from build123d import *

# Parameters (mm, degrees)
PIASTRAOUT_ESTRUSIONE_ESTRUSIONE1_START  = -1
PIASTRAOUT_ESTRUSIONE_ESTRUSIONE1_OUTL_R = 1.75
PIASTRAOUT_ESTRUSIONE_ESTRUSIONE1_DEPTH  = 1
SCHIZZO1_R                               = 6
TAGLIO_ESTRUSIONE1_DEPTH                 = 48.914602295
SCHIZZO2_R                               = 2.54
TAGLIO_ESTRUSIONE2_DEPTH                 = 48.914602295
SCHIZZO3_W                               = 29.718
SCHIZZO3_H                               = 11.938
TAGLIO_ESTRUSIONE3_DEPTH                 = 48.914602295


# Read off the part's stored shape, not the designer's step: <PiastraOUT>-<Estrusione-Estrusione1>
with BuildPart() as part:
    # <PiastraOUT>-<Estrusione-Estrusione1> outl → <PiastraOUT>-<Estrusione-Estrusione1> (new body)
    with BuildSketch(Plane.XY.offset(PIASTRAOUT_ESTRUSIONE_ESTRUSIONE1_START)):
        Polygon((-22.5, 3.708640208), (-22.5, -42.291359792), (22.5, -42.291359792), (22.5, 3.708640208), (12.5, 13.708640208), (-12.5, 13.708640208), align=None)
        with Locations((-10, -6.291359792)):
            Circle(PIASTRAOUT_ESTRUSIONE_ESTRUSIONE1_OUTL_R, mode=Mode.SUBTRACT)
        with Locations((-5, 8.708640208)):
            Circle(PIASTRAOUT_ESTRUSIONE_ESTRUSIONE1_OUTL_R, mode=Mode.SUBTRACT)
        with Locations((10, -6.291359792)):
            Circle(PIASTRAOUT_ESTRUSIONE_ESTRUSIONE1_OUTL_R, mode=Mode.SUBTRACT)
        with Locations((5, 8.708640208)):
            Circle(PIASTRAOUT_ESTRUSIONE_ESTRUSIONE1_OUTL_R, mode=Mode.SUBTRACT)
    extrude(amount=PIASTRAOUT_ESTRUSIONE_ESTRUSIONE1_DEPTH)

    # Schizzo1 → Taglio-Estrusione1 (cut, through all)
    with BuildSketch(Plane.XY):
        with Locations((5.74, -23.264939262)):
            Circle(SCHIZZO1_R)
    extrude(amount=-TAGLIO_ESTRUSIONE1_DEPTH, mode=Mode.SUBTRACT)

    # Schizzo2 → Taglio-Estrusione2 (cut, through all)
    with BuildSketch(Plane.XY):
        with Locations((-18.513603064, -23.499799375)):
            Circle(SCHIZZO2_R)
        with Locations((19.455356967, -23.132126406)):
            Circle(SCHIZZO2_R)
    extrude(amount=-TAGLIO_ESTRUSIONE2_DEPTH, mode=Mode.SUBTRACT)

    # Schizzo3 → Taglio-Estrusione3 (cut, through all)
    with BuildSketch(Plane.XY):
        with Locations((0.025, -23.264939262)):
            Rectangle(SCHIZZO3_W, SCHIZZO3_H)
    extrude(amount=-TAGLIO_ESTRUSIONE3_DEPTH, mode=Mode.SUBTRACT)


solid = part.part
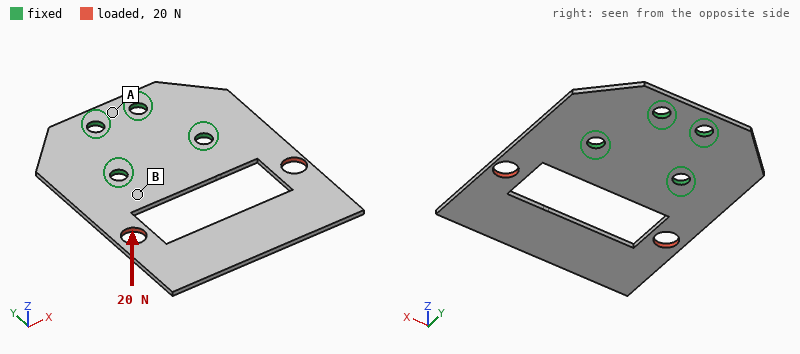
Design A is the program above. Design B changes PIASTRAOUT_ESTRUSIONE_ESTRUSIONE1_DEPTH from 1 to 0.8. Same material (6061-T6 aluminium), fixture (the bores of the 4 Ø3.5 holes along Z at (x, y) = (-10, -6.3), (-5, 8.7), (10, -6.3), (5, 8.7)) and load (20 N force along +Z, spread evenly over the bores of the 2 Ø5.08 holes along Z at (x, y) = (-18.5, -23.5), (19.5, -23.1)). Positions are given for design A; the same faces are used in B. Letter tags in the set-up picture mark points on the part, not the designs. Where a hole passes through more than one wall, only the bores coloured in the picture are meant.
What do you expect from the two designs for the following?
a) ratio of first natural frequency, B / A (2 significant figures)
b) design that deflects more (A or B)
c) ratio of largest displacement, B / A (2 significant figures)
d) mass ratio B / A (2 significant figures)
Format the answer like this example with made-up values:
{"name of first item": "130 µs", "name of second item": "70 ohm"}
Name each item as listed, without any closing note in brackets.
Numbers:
{"ratio of first natural frequency, B / A": "0.80", "design that deflects more": "B", "ratio of largest displacement, B / A": "1.9", "mass ratio B / A": "0.80"}
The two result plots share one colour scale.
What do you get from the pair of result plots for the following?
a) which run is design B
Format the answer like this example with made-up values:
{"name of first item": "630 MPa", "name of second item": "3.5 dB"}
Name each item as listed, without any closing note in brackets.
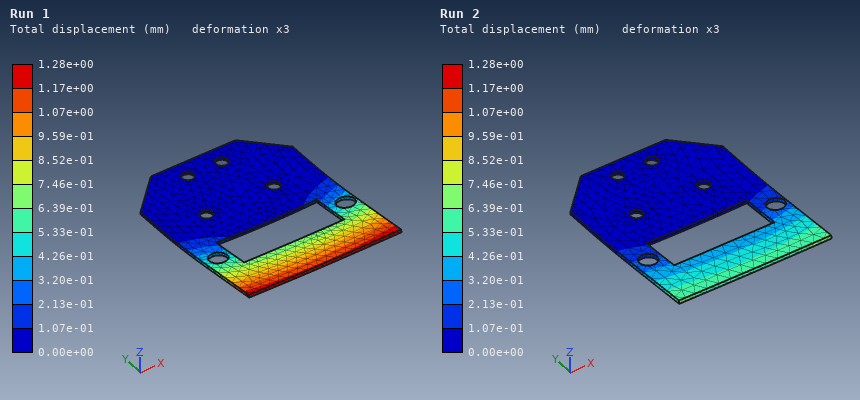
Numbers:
{"which run is design B": "Run 1"}
